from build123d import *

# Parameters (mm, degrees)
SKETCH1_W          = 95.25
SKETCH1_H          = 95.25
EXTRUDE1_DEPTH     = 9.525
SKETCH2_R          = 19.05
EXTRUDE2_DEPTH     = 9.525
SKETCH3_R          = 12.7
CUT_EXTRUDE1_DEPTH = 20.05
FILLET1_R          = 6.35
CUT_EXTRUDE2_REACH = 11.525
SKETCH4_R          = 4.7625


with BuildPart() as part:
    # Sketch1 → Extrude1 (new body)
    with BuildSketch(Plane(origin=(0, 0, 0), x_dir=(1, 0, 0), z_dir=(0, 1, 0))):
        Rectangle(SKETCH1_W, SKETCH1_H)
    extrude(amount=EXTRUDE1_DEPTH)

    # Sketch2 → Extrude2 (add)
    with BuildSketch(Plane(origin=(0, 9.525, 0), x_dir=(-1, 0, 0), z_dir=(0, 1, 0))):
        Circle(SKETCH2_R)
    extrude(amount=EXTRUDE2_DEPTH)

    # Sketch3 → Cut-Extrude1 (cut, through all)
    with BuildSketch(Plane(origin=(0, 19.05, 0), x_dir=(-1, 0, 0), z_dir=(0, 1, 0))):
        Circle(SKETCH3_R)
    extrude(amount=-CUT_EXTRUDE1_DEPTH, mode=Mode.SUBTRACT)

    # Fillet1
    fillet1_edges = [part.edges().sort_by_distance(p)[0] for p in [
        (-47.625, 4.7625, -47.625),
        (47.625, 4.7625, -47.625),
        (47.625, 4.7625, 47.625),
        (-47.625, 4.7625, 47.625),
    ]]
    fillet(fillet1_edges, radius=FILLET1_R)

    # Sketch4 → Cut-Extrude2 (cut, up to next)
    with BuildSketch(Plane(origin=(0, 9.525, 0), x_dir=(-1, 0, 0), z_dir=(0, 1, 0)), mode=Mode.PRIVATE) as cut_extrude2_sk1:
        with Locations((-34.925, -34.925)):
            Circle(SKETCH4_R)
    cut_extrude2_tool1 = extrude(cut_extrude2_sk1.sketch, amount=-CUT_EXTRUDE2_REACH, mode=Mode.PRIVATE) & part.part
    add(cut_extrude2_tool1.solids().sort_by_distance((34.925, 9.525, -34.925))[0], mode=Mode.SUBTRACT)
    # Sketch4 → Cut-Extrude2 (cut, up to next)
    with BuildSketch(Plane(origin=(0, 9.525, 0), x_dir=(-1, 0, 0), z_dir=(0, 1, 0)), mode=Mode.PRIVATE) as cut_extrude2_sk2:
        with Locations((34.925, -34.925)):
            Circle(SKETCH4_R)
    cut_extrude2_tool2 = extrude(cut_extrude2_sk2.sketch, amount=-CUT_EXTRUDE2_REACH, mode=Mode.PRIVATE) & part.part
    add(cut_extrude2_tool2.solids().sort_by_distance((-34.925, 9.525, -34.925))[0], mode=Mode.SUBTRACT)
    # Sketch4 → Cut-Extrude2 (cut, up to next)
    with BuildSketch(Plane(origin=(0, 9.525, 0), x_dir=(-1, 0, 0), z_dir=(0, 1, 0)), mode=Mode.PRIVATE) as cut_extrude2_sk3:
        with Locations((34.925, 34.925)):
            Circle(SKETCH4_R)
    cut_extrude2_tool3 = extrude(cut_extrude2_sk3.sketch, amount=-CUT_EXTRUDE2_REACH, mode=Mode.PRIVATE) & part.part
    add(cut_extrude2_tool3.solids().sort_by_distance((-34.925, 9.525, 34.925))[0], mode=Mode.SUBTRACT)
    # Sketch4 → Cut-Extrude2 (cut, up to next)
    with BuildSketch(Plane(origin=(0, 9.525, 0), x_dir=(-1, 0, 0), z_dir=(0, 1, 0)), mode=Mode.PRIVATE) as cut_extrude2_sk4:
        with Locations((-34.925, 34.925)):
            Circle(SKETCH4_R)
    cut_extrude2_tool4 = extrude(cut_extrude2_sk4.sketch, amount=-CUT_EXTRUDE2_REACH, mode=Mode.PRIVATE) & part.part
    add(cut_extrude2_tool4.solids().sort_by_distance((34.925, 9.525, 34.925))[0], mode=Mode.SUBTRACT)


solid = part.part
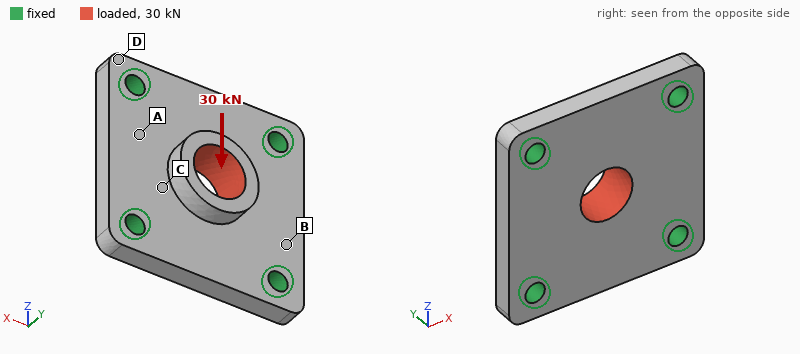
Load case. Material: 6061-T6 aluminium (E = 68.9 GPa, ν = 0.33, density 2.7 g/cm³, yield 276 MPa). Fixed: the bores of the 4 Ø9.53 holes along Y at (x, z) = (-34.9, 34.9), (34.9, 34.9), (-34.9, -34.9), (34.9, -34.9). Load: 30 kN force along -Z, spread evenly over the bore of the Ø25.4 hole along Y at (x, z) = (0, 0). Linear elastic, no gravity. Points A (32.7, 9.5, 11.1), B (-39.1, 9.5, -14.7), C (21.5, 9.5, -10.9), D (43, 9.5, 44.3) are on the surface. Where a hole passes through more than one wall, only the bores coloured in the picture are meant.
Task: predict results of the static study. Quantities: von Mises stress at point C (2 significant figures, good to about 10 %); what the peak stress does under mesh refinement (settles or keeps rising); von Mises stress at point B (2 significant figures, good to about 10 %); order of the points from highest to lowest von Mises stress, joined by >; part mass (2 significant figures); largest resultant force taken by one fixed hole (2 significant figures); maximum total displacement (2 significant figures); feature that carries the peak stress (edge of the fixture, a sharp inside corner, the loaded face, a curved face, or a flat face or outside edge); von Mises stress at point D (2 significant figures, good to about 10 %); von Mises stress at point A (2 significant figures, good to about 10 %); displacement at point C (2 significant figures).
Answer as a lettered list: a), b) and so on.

a) 53 MPa
b) keeps rising
c) 18 MPa
d) C > A > B > D
e) 230 g
f) 8.3 kN
g) 53 µm
h) edge of the fixture
i) 8.3 MPa
j) 29 MPa
k) 17 µm
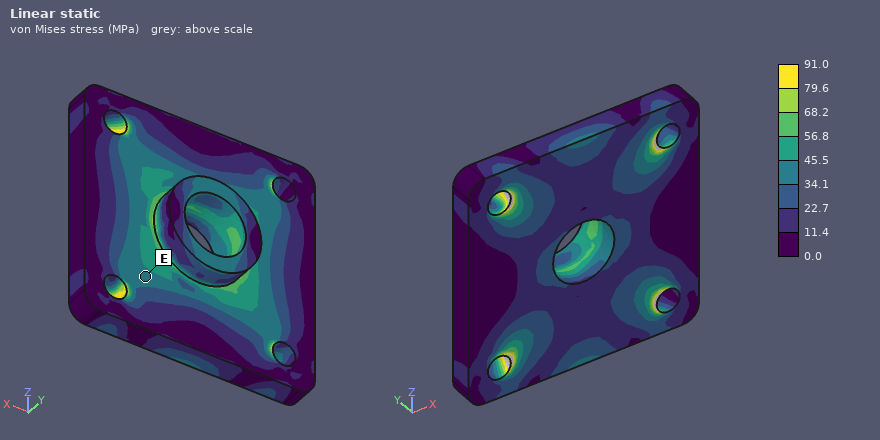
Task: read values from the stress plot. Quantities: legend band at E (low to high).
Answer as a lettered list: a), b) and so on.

a) 34.1 to 45.5 MPa
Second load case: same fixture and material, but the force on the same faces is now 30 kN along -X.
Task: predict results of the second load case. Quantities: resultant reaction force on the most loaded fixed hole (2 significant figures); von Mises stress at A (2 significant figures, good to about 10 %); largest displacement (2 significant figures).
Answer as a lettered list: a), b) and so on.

a) 8.3 kN
b) 22 MPa
c) 53 µm
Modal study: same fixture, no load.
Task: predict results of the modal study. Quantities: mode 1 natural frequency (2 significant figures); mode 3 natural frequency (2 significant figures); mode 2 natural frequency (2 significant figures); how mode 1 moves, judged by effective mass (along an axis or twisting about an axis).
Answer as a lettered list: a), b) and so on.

a) 7500 Hz
b) 11 kHz
c) 11 kHz
d) along Y
